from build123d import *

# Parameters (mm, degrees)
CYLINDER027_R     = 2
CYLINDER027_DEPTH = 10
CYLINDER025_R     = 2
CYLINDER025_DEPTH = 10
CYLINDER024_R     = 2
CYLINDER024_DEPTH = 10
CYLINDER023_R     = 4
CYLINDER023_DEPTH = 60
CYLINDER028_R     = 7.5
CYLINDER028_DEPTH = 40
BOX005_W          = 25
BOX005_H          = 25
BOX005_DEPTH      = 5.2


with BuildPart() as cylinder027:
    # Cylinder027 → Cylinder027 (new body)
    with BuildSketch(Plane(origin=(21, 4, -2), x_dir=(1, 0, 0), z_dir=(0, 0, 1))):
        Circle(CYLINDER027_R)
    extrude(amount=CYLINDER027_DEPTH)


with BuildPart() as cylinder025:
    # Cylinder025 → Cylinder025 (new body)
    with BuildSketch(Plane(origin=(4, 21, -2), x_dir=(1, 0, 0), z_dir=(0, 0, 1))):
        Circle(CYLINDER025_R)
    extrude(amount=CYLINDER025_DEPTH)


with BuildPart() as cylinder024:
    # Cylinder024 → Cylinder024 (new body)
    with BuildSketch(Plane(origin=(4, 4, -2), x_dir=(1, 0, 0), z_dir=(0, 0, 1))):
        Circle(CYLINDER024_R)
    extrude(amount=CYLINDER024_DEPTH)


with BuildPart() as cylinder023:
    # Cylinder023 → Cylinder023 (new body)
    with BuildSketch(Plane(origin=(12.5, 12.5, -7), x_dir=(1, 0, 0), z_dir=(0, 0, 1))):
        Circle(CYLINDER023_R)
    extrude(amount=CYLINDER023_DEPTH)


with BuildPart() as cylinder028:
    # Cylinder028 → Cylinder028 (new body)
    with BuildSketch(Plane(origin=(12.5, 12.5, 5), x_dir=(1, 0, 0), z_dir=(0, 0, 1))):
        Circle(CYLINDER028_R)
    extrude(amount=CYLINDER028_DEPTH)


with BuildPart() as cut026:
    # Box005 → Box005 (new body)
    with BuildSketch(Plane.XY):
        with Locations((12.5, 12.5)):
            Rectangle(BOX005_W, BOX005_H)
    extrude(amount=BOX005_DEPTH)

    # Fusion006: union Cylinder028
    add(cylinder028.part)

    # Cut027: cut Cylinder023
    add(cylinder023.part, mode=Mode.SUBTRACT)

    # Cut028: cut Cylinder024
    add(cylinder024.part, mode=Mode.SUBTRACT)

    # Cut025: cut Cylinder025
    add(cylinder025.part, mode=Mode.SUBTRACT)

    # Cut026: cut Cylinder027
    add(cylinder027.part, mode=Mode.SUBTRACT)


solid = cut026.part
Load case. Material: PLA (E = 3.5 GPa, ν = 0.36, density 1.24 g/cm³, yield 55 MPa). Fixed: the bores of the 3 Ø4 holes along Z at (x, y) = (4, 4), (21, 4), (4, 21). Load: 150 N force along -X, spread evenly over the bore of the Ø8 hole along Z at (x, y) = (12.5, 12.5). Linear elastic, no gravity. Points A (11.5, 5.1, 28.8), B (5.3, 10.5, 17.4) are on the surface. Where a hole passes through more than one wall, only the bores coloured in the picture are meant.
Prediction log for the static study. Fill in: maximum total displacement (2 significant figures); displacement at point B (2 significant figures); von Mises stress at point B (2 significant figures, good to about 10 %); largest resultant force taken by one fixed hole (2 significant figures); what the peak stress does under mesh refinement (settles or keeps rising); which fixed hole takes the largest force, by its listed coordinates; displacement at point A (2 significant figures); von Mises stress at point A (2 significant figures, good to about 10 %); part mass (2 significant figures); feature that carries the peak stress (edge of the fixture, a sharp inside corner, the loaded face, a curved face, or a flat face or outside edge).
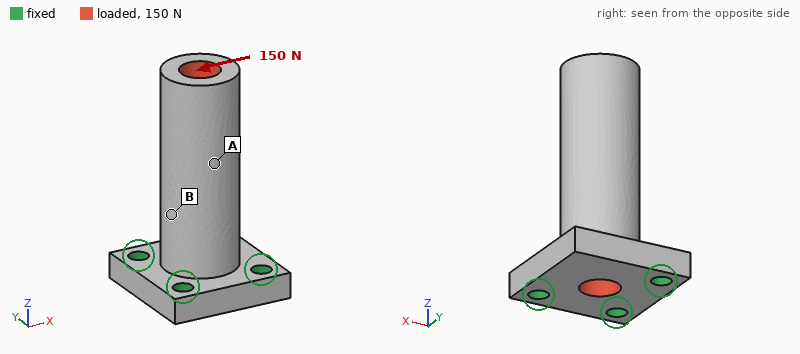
0.32 mm
0.097 mm
3.9 MPa
180 N
keeps rising
(21, 4)
0.18 mm
1.1 MPa
9.7 g
edge of the fixture
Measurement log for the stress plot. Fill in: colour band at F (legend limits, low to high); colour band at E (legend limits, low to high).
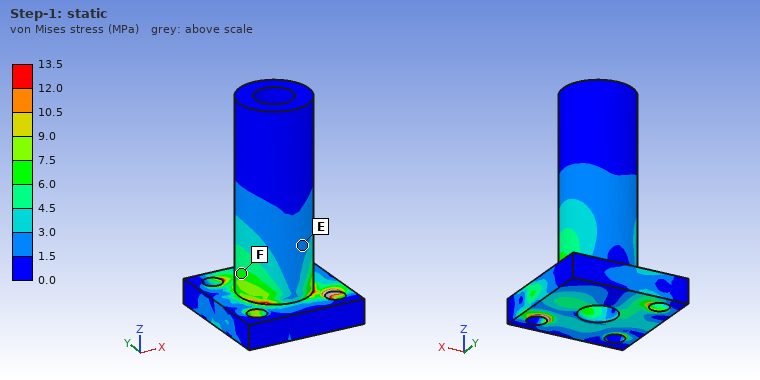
6.0 to 7.5 MPa
1.5 to 3.0 MPa
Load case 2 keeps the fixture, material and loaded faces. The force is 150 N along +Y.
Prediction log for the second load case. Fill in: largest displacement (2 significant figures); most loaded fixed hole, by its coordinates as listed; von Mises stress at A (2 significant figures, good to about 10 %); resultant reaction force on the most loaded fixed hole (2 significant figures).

0.32 mm
(4, 21)
1.4 MPa
180 N
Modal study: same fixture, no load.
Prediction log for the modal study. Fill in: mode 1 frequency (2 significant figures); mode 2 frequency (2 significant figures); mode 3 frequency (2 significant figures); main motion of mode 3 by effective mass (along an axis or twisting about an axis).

1400 Hz
1800 Hz
6000 Hz
twisting about Z
